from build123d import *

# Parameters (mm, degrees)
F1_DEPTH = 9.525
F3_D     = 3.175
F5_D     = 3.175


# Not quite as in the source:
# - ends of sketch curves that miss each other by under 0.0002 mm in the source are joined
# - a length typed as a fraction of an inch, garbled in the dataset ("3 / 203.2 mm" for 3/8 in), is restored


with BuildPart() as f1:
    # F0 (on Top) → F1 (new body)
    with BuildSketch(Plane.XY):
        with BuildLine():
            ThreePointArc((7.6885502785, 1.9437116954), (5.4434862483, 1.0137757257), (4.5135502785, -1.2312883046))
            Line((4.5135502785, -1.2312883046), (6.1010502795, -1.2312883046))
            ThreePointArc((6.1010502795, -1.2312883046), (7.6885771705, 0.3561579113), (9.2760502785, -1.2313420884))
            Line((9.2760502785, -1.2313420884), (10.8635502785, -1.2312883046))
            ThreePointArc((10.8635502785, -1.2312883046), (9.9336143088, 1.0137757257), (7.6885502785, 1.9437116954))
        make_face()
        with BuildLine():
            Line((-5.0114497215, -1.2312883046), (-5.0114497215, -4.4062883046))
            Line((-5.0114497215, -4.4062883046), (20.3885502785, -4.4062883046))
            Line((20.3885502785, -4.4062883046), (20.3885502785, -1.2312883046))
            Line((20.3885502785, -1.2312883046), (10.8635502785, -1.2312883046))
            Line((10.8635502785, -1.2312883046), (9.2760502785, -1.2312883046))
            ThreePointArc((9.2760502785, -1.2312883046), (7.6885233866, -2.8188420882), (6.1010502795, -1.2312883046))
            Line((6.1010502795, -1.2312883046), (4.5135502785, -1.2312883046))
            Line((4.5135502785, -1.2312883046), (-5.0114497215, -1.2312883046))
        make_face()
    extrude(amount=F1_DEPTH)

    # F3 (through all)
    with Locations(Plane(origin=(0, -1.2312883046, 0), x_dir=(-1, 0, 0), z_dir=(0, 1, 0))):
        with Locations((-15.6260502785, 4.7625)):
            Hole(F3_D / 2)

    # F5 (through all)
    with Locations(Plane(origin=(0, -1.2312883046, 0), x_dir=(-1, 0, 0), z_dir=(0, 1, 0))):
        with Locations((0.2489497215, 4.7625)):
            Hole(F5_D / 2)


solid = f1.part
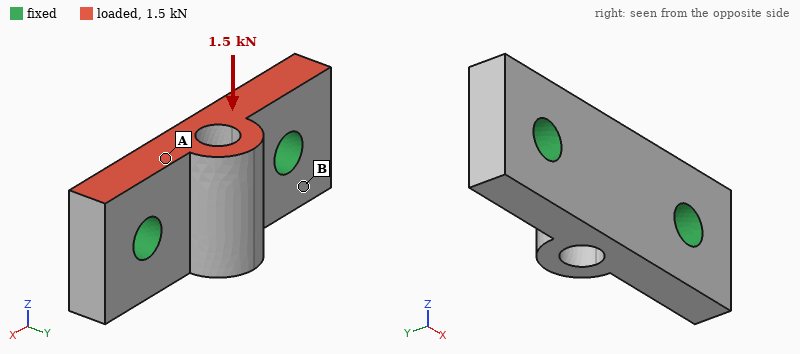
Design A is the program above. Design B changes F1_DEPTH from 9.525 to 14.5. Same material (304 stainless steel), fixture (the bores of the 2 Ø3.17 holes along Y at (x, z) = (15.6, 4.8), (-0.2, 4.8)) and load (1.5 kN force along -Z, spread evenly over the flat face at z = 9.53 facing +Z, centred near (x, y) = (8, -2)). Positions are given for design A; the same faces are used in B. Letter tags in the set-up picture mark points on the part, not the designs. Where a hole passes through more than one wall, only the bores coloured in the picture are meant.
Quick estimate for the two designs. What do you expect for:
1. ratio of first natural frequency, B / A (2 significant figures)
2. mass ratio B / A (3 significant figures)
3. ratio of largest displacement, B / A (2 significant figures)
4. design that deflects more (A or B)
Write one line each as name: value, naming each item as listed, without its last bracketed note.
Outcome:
ratio of first natural frequency, B / A: 0.50
mass ratio B / A: 1.56
ratio of largest displacement, B / A: 0.92
design that deflects more: A
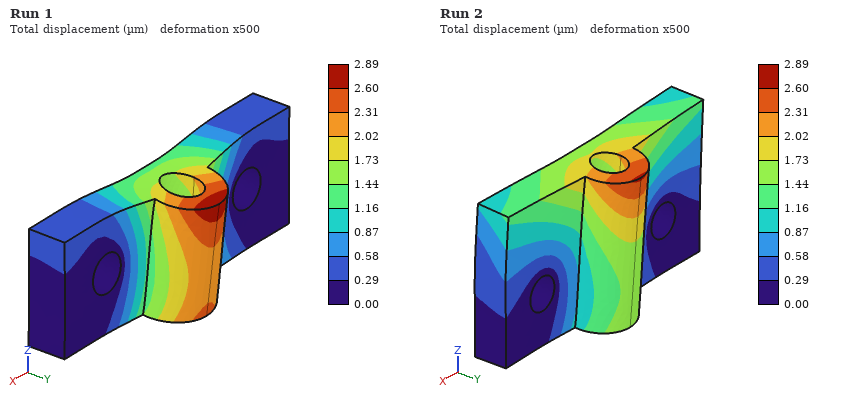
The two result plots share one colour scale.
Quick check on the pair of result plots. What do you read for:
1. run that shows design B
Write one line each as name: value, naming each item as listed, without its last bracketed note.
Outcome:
run that shows design B: Run 2
